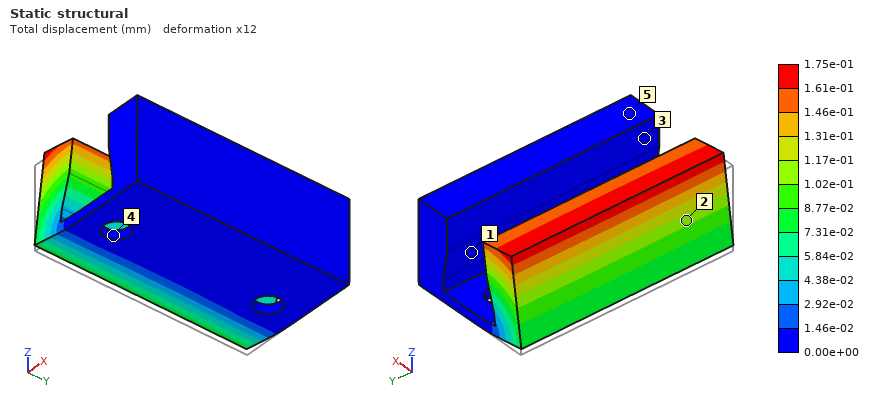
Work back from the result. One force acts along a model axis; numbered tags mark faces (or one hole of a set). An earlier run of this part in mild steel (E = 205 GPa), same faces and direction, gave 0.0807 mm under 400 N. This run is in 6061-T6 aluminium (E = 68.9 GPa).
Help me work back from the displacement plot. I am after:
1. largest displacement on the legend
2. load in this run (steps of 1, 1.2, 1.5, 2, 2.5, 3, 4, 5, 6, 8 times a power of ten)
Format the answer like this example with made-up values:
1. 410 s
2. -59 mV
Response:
1. 1.75e-01 mm
2. 300 N
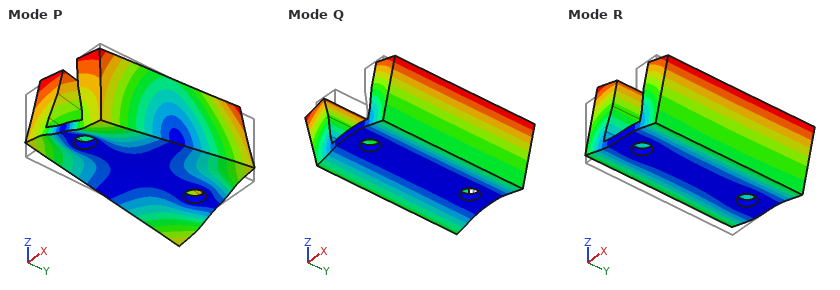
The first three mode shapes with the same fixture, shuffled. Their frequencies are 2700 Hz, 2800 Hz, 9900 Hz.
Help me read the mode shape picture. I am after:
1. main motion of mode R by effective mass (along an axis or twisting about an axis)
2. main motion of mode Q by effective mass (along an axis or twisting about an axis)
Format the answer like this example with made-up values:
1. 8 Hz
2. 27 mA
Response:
1. along X
2. along Z
